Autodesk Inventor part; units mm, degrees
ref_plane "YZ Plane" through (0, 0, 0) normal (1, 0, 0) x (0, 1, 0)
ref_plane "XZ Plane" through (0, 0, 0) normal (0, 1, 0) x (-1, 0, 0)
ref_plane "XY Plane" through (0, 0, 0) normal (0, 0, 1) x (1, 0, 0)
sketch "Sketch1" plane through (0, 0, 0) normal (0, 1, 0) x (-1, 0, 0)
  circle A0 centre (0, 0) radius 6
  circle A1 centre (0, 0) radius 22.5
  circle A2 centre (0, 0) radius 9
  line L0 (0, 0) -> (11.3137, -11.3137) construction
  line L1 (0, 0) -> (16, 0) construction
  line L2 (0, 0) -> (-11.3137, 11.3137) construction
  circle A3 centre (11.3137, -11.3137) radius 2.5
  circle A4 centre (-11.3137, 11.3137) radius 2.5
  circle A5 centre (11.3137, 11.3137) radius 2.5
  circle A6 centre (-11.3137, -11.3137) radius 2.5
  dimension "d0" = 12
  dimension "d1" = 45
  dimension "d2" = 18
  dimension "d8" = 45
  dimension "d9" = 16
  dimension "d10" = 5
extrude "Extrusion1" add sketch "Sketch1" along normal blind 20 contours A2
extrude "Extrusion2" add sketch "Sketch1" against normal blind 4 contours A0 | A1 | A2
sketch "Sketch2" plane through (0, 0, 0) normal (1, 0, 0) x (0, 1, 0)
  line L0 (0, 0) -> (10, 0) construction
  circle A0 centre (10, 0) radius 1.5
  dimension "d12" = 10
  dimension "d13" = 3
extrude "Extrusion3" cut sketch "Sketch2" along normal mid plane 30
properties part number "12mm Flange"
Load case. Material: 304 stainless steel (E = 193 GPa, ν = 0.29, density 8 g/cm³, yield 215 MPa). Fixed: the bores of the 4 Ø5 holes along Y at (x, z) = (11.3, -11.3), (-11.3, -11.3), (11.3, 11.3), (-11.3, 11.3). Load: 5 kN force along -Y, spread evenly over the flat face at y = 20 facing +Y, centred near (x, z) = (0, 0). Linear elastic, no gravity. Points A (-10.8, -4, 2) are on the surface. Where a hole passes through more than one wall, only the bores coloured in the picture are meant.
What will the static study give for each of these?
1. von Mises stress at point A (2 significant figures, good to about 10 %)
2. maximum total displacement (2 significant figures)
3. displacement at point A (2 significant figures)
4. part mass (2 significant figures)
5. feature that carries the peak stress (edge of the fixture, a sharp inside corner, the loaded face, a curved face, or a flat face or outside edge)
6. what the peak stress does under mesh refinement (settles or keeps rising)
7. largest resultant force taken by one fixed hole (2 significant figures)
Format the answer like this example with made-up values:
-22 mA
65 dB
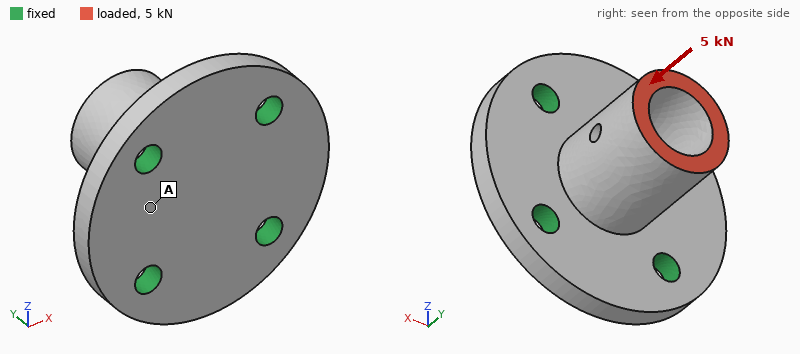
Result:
37 MPa
10 µm
4.4 µm
71 g
edge of the fixture
keeps rising
1.3 kN
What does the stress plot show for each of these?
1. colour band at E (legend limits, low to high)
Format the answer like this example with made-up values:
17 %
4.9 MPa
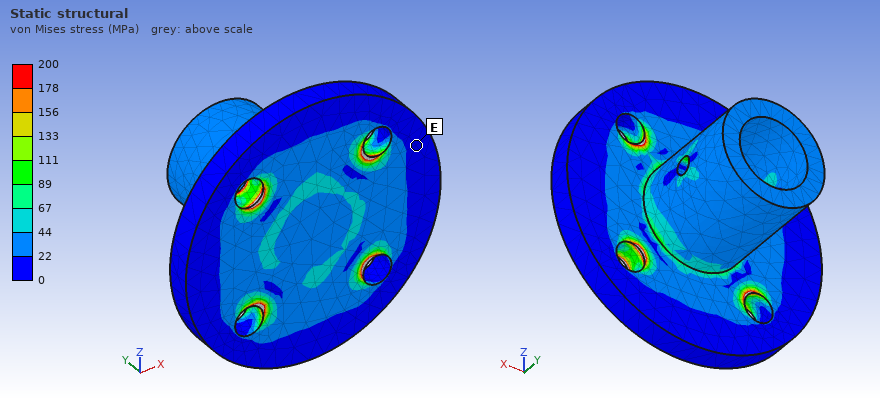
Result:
0 to 22 MPa
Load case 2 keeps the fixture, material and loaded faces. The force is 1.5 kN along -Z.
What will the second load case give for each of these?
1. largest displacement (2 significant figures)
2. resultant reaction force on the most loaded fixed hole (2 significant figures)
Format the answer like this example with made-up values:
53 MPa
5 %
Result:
25 µm
950 N
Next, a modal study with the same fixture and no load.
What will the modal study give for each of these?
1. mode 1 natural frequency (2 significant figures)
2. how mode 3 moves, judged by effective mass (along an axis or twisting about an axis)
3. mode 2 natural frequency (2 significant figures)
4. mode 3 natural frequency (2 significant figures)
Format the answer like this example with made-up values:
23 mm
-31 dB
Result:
14 kHz
along Y
14 kHz
23 kHz
